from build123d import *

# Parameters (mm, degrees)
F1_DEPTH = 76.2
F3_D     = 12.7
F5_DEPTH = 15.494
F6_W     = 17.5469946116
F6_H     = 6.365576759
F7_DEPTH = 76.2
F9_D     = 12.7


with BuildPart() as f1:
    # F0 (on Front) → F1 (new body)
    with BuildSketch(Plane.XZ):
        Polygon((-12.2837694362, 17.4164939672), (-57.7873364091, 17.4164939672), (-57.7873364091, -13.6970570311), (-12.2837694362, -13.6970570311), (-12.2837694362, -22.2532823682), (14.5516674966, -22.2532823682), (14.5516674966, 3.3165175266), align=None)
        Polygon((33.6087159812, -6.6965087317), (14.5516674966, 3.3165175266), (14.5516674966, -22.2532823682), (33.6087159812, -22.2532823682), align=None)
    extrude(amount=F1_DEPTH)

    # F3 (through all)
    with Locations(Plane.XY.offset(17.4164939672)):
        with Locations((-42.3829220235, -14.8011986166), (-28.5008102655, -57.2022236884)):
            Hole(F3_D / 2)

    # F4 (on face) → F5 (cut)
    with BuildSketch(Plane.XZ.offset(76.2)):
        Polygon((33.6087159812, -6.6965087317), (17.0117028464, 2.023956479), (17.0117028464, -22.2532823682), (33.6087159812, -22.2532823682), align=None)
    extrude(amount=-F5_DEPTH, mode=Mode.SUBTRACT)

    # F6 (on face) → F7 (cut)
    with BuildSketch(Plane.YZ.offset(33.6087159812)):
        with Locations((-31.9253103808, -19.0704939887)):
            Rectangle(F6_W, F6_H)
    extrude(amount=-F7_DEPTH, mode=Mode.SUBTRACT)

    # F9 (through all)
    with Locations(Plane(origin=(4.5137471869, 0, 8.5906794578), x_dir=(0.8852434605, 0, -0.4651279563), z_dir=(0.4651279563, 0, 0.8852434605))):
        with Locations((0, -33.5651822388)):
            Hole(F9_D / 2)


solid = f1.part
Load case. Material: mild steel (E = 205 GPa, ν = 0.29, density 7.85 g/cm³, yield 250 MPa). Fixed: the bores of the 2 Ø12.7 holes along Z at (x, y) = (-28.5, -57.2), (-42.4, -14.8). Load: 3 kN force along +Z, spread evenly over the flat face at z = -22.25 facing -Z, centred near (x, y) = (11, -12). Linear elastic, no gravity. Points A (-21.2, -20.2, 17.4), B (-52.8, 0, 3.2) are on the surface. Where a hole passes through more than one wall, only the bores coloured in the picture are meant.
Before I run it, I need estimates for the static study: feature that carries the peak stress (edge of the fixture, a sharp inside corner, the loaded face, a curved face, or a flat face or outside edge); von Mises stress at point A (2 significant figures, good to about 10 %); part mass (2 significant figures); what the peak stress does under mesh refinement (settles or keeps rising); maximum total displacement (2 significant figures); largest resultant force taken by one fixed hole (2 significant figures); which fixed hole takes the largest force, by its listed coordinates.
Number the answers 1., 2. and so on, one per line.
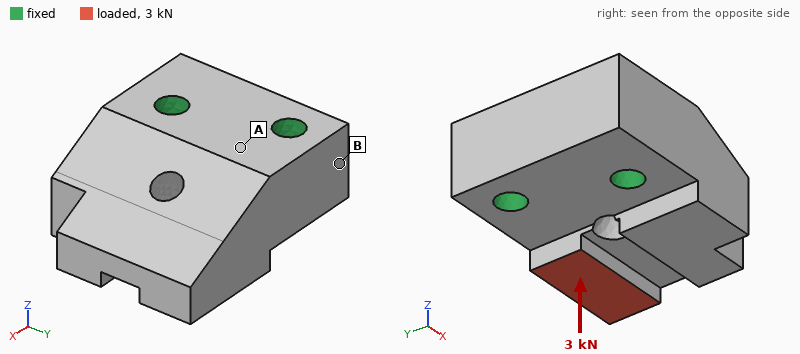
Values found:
1. edge of the fixture
2. 9.4 MPa
3. 1.4 kg
4. keeps rising
5. 12 µm
6. 1.9 kN
7. (-42.4, -14.8)
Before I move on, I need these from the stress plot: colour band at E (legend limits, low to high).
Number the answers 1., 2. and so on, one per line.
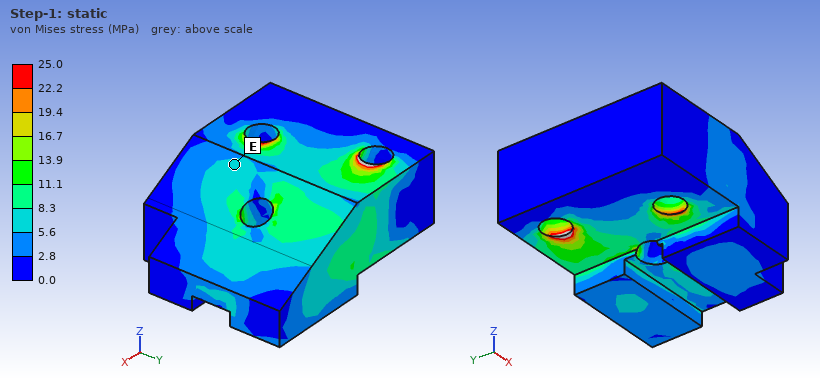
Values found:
1. 5.6 to 8.3 MPa
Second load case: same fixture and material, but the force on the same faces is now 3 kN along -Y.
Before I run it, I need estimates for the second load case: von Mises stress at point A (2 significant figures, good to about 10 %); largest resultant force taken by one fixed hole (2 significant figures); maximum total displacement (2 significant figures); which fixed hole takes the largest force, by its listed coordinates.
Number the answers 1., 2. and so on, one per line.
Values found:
1. 3.5 MPa
2. 3.5 kN
3. 6.2 µm
4. (-28.5, -57.2)
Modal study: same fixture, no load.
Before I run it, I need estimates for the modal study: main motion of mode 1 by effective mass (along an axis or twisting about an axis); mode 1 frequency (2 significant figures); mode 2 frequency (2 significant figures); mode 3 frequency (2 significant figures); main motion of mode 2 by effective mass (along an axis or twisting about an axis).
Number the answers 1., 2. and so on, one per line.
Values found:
1. along Z
2. 5800 Hz
3. 8800 Hz
4. 10 kHz
5. along Y
